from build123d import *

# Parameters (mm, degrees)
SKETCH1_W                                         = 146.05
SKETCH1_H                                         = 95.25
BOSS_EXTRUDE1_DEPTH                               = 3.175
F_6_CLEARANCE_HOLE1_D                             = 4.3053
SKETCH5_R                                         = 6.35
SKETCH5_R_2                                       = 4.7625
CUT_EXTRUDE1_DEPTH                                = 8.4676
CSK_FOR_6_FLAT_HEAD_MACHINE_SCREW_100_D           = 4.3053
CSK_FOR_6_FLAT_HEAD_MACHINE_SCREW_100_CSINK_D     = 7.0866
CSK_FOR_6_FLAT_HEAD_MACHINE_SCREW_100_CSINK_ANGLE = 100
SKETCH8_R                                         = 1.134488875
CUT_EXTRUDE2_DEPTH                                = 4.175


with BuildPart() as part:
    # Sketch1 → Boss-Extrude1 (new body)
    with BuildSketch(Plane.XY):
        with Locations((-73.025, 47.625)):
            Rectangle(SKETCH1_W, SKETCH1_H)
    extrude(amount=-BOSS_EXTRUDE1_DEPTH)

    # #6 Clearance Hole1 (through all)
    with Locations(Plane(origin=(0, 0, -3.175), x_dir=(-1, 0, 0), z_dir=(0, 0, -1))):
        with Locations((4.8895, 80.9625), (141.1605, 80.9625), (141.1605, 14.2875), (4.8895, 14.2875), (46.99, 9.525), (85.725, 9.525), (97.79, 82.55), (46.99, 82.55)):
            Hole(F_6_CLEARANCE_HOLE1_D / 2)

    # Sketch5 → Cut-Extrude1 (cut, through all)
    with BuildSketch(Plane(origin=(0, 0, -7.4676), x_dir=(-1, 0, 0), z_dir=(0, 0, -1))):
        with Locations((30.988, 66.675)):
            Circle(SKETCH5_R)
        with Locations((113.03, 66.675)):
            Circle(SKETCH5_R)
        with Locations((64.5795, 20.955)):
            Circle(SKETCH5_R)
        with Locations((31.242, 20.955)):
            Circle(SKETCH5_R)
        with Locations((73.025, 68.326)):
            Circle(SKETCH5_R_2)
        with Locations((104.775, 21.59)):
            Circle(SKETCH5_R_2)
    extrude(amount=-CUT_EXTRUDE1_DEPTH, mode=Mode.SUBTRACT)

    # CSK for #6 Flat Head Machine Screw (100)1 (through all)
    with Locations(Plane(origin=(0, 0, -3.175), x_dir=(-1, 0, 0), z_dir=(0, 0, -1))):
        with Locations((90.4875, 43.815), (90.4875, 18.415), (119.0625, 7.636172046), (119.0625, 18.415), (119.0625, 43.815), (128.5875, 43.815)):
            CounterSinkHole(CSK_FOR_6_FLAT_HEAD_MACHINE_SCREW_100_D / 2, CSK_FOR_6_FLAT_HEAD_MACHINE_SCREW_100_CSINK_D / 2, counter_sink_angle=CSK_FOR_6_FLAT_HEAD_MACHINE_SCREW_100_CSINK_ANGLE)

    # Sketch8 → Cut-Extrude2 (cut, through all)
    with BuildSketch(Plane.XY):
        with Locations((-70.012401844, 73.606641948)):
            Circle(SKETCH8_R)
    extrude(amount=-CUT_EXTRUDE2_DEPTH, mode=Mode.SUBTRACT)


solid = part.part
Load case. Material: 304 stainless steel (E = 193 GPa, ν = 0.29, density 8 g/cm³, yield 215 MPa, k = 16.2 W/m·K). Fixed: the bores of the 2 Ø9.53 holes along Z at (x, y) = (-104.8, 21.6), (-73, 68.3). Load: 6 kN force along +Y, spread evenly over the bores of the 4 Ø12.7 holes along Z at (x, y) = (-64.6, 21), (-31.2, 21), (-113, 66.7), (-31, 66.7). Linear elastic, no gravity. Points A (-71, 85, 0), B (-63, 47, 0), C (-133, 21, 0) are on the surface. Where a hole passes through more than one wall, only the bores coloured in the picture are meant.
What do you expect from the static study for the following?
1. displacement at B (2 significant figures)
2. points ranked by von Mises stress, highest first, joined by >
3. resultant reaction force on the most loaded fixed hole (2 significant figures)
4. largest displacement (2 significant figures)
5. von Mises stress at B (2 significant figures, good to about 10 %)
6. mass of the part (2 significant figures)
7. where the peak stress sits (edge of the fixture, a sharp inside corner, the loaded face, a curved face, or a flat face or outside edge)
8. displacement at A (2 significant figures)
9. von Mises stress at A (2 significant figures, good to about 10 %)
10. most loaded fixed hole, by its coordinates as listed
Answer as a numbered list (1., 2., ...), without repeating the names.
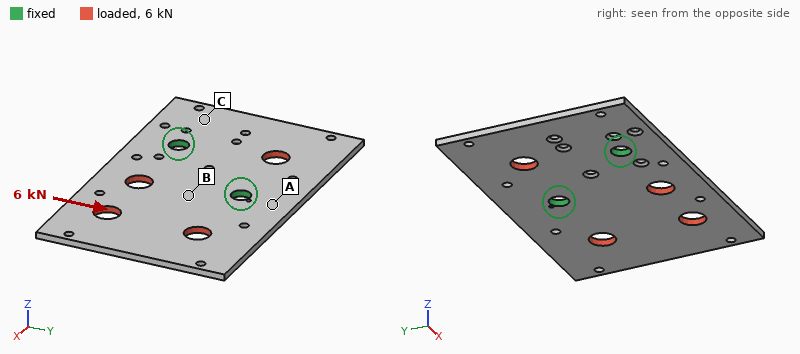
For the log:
1. 6.5 µm
2. B > A > C
3. 5.2 kN
4. 26 µm
5. 40 MPa
6. 330 g
7. edge of the fixture
8. 4.5 µm
9. 23 MPa
10. (-73, 68.3)
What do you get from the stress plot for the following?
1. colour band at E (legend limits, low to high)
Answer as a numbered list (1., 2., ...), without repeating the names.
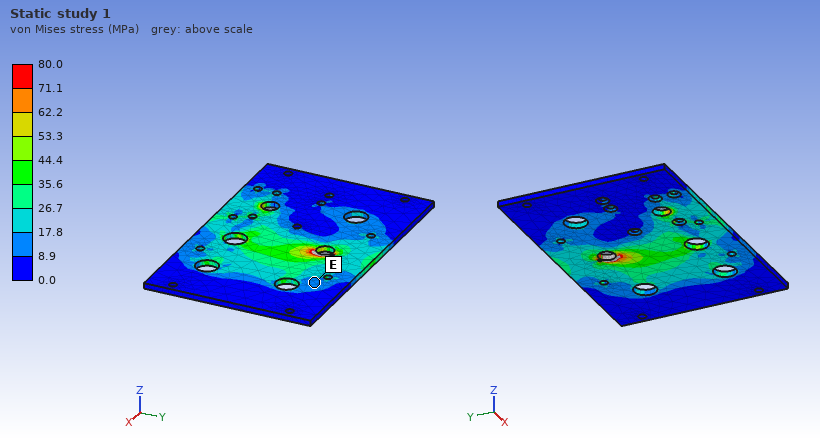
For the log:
1. 8.9 to 17.8 MPa
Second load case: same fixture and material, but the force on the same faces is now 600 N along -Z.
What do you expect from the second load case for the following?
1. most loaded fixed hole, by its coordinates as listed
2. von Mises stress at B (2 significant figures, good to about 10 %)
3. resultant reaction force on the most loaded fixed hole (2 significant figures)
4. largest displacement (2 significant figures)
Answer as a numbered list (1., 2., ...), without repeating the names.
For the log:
1. (-73, 68.3)
2. 67 MPa
3. 430 N
4. 0.75 mm
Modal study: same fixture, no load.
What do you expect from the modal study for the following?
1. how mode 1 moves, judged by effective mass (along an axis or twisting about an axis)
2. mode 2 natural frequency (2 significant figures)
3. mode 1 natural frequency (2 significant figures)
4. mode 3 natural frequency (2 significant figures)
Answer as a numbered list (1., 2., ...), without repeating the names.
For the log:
1. along Z
2. 760 Hz
3. 390 Hz
4. 780 Hz
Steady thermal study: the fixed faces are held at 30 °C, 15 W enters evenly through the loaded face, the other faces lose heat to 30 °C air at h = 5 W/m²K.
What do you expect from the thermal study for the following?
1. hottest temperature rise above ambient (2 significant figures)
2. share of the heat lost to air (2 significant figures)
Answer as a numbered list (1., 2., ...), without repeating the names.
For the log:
1. 89 K
2. 38 %
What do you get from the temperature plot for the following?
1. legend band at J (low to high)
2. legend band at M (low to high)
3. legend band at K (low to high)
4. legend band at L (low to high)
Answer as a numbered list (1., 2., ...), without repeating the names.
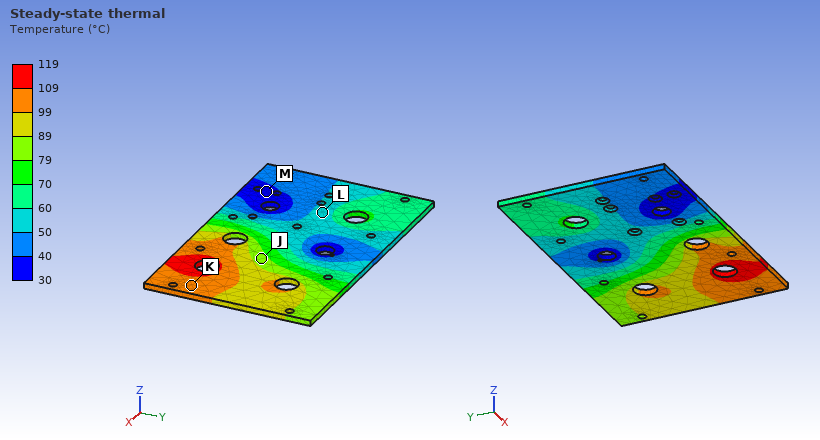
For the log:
1. 79 to 89 °C
2. 30 to 40 °C
3. 99 to 109 °C
4. 50 to 60 °C
